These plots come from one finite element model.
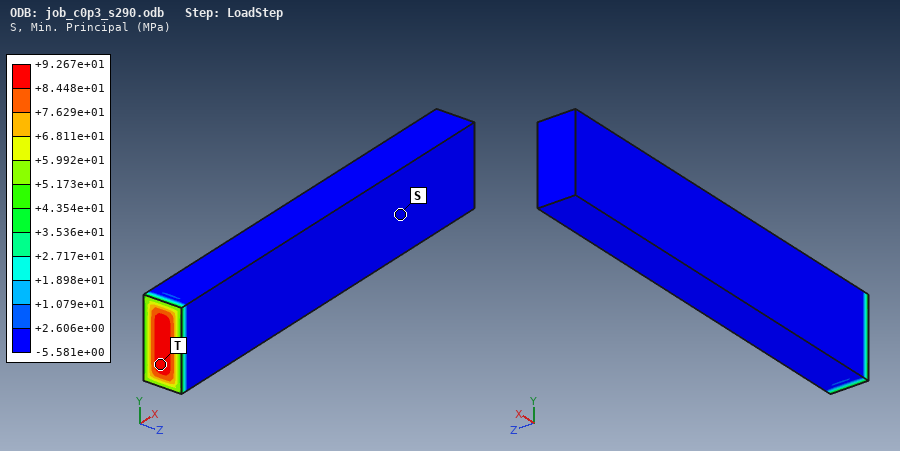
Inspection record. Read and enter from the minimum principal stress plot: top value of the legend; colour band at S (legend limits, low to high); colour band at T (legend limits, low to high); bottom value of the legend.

+9.267e+01 MPa
-5.581e+00 to +2.606e+00 MPa
+8.448e+01 to +9.267e+01 MPa
-5.581e+00 MPa
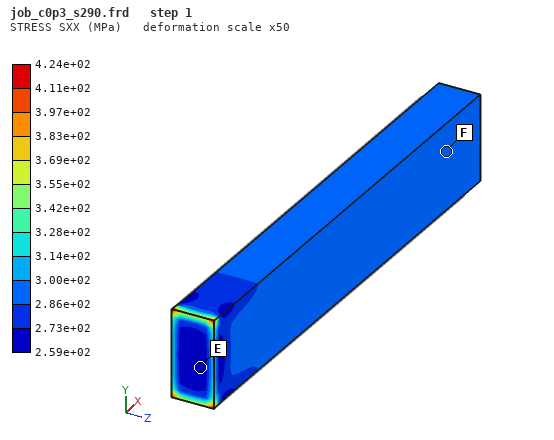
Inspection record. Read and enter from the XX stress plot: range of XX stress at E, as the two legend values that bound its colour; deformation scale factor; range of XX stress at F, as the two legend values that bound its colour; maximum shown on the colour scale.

2.59e+02 to 2.73e+02 MPa
50
2.86e+02 to 3.00e+02 MPa
4.24e+02 MPa
